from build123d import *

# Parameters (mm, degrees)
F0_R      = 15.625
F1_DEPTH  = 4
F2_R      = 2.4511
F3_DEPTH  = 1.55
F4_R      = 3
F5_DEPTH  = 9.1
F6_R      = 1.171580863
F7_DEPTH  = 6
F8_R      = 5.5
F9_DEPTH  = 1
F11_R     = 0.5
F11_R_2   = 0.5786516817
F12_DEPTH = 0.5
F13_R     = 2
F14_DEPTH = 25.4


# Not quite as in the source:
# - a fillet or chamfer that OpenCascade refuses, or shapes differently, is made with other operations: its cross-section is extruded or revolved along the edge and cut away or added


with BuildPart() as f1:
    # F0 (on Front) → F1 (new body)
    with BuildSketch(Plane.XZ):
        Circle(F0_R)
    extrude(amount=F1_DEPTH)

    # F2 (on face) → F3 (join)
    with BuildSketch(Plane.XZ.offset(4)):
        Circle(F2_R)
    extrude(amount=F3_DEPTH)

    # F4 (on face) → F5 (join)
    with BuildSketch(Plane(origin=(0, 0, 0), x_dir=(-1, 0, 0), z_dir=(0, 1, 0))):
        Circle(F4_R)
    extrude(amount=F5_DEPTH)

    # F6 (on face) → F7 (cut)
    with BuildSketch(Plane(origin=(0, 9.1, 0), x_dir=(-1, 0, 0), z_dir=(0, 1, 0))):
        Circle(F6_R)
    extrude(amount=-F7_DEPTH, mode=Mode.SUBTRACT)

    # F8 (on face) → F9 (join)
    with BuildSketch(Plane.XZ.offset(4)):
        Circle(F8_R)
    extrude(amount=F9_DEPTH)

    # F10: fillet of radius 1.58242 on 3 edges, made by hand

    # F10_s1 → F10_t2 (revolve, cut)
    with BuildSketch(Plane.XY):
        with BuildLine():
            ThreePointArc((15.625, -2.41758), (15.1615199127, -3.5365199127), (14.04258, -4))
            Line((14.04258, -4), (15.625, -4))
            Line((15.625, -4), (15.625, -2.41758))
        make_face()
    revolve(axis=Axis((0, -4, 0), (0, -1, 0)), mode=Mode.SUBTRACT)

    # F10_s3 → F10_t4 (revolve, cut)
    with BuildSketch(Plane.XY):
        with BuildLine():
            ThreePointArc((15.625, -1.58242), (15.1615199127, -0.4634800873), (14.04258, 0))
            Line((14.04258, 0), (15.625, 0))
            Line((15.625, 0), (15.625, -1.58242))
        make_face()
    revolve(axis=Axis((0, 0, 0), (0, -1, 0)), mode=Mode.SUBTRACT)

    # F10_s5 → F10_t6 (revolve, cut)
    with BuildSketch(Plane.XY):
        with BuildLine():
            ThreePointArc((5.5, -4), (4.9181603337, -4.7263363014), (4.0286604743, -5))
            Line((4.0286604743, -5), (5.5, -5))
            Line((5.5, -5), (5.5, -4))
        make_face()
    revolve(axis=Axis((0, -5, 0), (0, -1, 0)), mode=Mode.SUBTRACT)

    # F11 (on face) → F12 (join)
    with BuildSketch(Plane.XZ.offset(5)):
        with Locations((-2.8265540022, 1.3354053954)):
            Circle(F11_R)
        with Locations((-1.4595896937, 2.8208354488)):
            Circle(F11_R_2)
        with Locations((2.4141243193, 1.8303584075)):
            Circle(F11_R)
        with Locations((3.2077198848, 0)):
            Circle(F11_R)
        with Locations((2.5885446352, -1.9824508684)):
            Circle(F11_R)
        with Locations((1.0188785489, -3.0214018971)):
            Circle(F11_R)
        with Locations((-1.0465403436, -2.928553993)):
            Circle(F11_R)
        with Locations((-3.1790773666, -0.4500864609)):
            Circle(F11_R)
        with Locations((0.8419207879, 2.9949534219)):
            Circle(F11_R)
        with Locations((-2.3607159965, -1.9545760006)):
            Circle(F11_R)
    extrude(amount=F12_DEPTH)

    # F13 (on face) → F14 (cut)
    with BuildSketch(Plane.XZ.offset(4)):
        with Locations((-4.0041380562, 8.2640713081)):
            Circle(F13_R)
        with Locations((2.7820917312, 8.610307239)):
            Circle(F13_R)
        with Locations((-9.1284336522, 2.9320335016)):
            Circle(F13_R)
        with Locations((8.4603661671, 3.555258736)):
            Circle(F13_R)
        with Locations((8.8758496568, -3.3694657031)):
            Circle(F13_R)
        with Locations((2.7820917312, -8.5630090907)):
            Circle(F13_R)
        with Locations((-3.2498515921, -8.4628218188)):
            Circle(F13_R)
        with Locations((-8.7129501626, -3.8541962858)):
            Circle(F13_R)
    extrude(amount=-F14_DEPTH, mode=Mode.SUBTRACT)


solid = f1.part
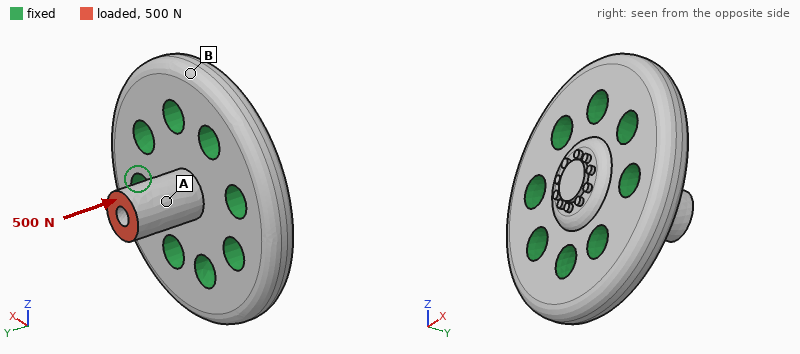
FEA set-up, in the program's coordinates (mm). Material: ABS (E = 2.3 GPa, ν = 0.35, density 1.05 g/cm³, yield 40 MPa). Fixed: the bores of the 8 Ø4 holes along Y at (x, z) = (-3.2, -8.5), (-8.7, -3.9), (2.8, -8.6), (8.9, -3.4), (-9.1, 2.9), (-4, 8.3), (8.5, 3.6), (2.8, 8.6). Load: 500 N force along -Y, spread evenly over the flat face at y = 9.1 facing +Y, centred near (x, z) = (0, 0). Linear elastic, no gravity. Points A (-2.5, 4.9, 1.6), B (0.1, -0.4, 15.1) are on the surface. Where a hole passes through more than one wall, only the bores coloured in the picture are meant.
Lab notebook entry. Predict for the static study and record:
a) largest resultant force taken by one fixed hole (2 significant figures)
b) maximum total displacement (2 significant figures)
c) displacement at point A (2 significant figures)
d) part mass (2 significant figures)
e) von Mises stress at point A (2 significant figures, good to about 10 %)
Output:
70 N
0.12 mm
0.083 mm
3.0 g
20 MPa
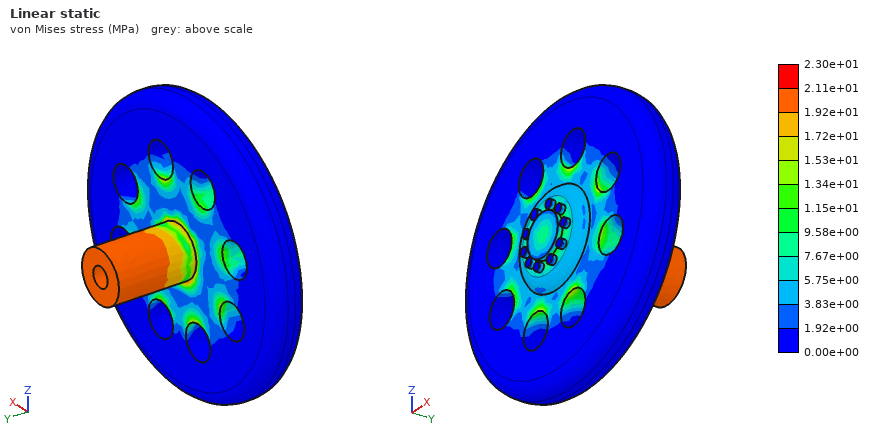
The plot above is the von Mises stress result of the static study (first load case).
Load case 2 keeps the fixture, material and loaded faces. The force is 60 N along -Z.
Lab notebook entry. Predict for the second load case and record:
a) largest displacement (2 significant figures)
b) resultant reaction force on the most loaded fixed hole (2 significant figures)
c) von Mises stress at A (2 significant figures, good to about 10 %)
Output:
0.21 mm
30 N
8.5 MPa
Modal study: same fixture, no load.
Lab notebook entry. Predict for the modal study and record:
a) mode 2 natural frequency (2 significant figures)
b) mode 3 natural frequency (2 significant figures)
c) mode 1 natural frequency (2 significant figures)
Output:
10 kHz
23 kHz
10 kHz
